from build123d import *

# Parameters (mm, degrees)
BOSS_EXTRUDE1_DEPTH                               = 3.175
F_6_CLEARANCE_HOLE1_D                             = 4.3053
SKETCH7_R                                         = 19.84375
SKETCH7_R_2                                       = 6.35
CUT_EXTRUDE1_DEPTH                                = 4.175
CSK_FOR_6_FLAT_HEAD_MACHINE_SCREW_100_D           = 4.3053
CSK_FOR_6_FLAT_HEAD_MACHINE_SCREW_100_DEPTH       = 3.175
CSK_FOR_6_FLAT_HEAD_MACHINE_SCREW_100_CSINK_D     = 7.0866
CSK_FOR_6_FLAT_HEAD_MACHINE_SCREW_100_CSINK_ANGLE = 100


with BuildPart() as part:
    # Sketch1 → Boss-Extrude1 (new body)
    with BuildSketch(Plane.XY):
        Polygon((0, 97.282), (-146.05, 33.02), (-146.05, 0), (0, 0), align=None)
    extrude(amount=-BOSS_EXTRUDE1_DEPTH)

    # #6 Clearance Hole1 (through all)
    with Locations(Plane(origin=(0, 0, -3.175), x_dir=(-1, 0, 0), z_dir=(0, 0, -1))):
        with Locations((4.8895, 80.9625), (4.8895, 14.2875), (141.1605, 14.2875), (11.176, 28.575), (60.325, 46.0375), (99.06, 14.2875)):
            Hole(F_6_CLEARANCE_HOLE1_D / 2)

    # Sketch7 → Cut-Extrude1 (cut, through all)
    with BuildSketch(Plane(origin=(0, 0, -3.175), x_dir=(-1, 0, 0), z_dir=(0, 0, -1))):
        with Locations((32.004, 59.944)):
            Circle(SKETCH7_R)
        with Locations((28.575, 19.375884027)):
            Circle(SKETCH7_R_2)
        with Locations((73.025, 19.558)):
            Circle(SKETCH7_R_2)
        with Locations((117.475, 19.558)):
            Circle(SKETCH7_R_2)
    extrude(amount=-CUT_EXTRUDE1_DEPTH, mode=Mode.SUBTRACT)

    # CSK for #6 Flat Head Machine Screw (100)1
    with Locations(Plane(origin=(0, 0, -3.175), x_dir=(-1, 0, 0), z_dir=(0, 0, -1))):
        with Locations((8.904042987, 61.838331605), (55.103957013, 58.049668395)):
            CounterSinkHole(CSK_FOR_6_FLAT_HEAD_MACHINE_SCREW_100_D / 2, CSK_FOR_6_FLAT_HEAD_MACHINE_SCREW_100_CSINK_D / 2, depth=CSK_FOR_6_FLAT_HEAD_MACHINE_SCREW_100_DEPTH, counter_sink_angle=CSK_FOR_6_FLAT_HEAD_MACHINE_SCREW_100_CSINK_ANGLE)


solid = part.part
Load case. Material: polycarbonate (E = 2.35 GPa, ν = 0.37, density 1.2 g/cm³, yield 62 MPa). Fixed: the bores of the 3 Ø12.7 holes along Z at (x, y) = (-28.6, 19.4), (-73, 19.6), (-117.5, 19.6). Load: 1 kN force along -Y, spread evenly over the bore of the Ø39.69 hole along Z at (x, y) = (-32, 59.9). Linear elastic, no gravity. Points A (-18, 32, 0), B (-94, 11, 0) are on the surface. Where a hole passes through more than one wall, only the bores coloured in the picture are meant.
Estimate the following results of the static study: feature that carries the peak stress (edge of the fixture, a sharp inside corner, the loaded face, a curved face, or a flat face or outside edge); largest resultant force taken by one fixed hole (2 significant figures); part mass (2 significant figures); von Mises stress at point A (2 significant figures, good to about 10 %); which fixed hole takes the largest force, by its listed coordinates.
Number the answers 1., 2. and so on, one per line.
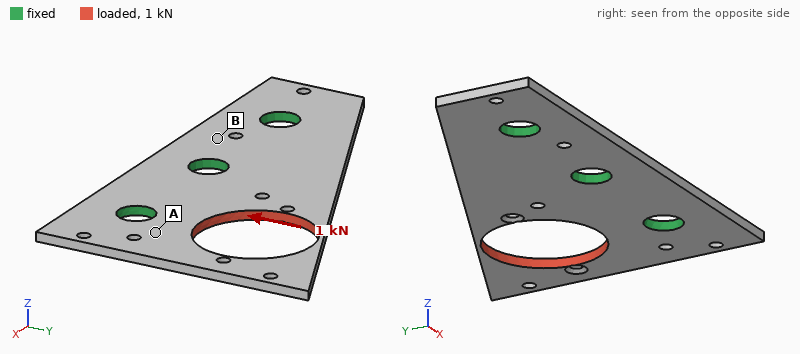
1. a curved face
2. 810 N
3. 30 g
4. 7.8 MPa
5. (-28.6, 19.4)
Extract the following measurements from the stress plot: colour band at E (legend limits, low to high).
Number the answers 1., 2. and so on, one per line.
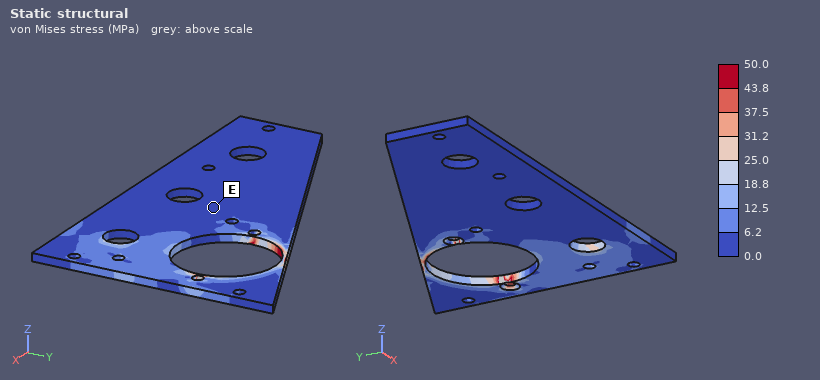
1. 0.0 to 6.2 MPa
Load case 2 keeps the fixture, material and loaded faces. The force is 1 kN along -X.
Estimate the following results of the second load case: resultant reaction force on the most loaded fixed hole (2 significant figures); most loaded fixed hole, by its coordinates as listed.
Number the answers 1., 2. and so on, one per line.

1. 660 N
2. (-28.6, 19.4)
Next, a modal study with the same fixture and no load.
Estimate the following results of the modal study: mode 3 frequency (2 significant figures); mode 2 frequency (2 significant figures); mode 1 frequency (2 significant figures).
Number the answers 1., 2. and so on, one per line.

1. 720 Hz
2. 480 Hz
3. 170 Hz
